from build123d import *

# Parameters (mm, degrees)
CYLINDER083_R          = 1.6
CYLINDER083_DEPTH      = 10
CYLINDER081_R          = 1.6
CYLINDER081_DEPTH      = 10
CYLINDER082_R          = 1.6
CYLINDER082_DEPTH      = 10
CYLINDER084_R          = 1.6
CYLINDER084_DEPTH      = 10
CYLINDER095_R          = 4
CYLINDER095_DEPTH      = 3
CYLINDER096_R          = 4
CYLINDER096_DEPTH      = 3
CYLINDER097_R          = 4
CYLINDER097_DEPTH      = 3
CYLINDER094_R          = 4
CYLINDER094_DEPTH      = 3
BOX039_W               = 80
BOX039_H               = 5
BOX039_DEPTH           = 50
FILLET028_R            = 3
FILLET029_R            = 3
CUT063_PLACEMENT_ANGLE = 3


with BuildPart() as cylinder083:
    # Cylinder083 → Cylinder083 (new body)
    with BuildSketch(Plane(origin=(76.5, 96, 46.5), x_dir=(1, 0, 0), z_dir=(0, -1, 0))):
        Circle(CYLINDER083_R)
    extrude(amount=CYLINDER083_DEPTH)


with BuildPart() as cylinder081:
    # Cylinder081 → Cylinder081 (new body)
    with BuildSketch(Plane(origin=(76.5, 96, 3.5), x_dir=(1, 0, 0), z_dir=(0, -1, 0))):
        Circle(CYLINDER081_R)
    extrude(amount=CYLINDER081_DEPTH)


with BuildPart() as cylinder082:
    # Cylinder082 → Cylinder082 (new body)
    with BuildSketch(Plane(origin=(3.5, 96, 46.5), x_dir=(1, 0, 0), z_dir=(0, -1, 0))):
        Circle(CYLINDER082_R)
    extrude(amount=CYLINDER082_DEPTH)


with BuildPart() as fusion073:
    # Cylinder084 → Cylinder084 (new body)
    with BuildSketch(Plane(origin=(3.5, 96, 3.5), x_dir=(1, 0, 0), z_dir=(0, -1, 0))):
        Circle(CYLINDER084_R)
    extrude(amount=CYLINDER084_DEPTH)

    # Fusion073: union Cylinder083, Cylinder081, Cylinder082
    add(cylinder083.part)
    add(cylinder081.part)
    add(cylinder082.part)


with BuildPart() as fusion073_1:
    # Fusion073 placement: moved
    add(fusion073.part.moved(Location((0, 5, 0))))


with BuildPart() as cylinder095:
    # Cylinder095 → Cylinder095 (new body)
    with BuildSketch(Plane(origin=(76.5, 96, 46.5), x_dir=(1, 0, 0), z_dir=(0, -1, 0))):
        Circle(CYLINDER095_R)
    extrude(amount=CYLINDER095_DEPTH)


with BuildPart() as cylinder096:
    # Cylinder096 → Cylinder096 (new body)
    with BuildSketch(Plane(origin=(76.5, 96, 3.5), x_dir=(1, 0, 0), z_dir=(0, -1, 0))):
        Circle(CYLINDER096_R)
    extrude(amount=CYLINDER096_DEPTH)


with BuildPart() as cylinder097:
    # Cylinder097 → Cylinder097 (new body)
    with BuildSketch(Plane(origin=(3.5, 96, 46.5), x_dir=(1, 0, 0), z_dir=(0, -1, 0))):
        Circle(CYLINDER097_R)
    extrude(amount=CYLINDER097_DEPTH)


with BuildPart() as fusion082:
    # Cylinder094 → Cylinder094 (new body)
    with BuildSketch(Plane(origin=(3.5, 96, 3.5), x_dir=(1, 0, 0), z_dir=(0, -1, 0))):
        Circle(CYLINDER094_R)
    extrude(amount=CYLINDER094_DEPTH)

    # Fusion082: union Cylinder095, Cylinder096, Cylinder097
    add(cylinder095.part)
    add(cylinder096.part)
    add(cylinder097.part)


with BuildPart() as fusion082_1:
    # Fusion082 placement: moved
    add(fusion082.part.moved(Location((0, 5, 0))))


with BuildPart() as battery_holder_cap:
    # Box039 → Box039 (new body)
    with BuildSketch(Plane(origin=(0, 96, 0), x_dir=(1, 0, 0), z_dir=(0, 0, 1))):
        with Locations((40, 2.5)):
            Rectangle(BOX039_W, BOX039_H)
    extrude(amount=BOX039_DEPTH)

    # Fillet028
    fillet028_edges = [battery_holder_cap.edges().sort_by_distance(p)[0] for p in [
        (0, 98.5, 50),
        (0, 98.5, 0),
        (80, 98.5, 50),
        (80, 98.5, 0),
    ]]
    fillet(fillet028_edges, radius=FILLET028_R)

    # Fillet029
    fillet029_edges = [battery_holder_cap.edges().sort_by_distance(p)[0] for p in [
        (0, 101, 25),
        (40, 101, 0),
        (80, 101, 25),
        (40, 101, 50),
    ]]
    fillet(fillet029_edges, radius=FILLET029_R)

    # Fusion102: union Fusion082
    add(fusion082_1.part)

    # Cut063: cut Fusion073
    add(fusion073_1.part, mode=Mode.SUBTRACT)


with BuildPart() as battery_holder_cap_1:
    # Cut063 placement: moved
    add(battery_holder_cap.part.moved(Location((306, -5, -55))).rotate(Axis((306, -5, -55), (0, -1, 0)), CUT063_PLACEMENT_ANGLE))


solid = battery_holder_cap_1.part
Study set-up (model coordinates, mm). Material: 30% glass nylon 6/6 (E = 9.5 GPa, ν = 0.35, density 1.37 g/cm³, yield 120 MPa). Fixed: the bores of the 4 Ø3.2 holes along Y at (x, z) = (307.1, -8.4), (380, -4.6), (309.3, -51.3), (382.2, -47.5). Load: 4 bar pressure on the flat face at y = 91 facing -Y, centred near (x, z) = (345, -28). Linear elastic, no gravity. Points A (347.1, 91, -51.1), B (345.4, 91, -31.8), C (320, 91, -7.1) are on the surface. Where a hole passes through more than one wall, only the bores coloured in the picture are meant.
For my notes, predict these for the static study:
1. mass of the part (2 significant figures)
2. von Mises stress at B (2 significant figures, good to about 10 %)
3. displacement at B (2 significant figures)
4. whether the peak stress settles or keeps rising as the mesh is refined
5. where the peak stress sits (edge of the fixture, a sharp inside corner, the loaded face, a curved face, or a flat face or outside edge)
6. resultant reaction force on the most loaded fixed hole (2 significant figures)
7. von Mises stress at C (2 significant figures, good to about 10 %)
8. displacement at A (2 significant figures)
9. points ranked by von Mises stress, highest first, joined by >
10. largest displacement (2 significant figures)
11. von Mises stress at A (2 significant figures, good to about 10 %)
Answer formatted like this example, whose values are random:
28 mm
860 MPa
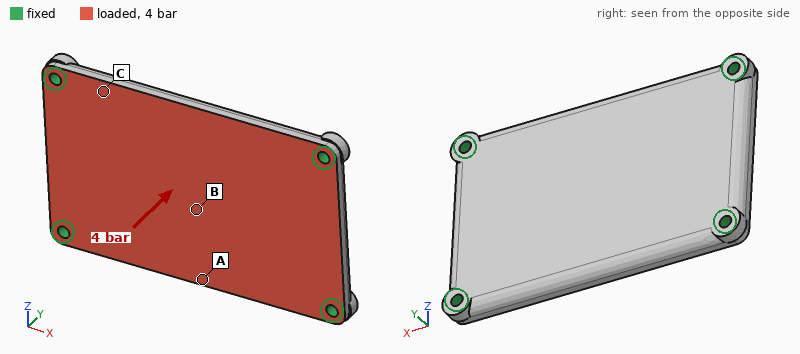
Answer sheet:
27 g
24 MPa
0.49 mm
keeps rising
edge of the fixture
400 N
9.8 MPa
0.49 mm
A > B > C
0.50 mm
30 MPa
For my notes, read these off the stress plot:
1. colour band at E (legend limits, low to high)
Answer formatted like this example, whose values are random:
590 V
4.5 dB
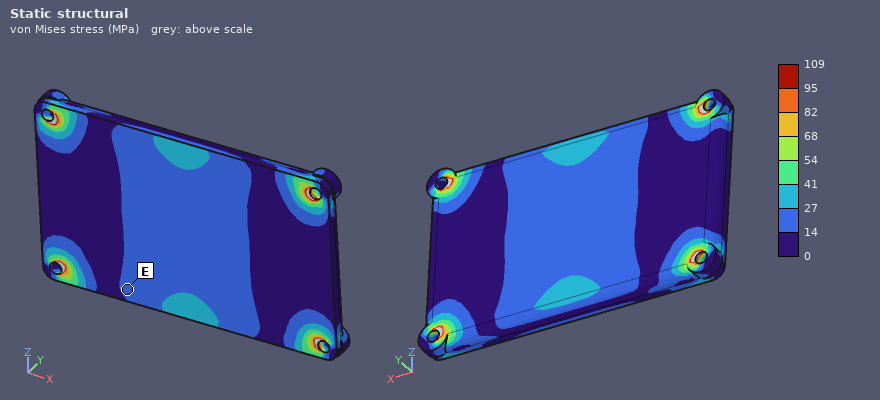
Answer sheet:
14 to 27 MPa
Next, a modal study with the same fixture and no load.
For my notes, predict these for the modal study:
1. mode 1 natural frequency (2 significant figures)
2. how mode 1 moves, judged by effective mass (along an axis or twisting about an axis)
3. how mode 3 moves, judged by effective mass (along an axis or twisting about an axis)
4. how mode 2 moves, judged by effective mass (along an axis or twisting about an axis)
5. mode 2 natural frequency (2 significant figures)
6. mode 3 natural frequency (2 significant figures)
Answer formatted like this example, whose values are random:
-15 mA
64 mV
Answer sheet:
2000 Hz
along Y
twisting about Z
twisting about X
3300 Hz
5100 Hz
